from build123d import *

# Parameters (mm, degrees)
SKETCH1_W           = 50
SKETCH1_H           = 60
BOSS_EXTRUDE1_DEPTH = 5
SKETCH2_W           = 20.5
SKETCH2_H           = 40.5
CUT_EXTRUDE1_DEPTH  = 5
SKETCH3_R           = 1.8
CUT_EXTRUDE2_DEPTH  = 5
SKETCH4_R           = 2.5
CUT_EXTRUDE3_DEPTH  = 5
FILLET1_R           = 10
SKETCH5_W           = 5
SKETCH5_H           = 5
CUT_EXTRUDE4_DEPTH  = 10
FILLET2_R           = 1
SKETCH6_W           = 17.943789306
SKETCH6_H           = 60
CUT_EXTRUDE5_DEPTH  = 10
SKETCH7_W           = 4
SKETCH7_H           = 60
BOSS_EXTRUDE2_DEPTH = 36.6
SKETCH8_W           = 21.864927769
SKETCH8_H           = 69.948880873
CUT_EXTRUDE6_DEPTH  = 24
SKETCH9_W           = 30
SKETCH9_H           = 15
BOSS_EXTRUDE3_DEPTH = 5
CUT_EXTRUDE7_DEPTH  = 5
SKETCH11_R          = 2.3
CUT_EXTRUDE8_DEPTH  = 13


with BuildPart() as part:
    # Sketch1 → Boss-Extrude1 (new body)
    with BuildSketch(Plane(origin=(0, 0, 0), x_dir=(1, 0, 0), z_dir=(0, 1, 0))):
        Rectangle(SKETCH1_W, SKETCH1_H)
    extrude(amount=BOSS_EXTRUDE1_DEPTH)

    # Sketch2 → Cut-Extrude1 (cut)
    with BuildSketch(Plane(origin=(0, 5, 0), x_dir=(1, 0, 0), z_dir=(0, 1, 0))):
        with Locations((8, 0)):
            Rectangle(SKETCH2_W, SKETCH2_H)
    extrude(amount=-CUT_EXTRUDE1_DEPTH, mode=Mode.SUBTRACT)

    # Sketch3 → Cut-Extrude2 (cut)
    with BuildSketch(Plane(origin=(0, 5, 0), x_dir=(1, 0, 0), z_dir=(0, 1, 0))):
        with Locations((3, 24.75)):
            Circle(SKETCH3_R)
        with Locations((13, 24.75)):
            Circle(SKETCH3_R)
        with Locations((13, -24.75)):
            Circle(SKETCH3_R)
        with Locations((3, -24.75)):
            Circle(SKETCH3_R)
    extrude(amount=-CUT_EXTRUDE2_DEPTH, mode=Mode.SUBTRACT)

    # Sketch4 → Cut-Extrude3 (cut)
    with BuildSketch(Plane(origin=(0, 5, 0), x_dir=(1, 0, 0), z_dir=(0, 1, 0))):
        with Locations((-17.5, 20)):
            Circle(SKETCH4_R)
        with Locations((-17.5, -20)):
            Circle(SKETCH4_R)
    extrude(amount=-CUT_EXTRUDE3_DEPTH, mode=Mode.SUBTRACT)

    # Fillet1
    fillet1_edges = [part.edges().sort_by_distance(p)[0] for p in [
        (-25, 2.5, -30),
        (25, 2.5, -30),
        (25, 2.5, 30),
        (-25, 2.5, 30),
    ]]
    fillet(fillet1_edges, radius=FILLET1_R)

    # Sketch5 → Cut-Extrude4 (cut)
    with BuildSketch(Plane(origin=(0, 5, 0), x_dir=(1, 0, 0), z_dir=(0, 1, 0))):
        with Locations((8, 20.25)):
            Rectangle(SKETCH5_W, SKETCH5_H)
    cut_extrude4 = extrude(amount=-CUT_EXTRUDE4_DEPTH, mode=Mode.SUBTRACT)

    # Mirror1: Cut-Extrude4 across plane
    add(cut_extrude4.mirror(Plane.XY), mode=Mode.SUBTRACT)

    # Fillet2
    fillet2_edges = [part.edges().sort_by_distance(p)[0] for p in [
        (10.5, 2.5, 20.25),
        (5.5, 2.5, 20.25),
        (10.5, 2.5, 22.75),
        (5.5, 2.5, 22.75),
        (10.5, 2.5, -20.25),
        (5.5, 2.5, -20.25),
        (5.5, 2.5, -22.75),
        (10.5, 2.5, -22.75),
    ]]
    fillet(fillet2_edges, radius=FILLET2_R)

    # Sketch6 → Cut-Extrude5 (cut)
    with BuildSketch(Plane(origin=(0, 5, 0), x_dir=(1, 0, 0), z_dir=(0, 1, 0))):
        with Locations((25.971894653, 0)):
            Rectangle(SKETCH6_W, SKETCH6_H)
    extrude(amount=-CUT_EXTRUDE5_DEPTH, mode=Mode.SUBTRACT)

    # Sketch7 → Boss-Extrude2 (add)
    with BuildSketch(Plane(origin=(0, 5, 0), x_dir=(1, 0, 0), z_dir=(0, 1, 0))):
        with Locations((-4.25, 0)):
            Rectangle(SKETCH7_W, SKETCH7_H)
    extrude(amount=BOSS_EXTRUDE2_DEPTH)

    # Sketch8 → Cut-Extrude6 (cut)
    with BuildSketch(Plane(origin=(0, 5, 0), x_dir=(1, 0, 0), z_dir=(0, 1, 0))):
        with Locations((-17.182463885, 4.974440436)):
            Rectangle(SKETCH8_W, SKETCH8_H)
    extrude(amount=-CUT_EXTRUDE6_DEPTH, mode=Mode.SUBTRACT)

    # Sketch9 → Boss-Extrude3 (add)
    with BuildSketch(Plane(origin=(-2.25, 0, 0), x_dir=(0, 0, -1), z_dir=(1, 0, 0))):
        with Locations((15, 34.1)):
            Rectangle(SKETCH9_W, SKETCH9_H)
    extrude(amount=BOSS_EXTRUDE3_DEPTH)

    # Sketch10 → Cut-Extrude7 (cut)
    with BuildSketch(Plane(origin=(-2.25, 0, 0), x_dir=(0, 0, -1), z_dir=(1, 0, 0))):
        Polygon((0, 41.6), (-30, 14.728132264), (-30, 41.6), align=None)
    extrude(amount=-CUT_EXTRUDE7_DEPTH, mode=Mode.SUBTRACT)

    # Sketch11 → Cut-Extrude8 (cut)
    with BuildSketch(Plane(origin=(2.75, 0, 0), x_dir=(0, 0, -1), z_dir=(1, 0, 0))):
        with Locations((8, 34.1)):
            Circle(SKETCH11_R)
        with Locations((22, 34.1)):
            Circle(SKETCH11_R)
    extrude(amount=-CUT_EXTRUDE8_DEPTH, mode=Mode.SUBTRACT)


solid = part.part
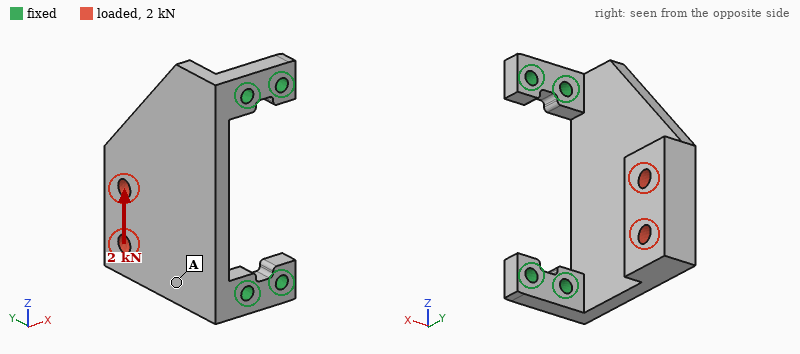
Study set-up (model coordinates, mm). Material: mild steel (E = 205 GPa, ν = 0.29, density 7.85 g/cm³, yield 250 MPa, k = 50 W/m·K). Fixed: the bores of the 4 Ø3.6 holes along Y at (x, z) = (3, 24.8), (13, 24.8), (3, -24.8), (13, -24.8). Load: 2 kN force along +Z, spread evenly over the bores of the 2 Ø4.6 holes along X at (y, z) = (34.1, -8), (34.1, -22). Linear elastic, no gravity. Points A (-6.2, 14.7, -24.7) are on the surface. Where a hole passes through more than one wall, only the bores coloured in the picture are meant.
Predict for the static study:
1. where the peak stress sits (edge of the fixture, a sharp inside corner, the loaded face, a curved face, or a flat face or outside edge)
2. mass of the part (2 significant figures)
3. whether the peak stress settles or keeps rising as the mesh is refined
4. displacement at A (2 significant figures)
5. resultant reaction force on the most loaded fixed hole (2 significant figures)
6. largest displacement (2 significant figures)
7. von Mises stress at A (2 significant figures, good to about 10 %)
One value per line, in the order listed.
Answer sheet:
edge of the fixture
93 g
keeps rising
19 µm
1.8 kN
50 µm
35 MPa
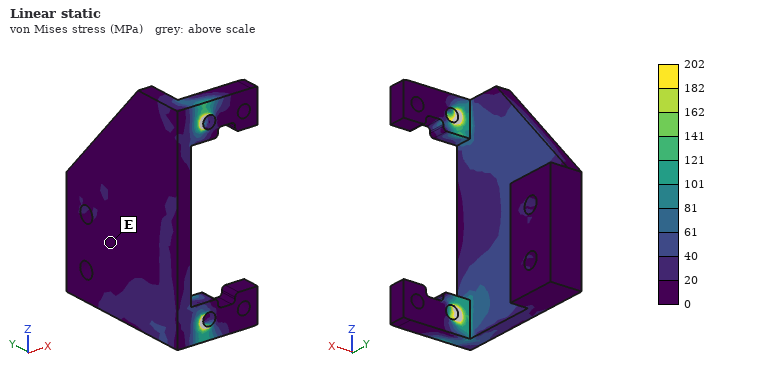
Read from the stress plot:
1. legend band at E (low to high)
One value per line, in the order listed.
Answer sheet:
0 to 20 MPa
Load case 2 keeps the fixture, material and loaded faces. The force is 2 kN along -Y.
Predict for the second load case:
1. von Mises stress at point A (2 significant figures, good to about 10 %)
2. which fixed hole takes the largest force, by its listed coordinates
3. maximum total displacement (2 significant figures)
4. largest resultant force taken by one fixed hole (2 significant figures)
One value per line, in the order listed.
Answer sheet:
26 MPa
(3, -24.8)
64 µm
1.7 kN
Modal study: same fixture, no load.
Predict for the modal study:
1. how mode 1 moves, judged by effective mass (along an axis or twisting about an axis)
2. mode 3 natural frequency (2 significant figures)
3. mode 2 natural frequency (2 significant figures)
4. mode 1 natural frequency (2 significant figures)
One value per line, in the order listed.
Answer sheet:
along X
7000 Hz
4400 Hz
1200 Hz
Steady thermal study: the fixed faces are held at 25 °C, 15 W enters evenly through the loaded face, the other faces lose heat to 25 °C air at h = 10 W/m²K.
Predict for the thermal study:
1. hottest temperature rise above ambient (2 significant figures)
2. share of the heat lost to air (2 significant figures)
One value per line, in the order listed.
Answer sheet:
75 K
16 %
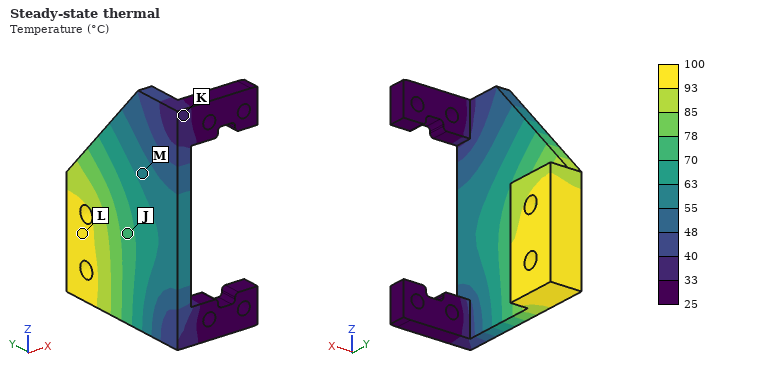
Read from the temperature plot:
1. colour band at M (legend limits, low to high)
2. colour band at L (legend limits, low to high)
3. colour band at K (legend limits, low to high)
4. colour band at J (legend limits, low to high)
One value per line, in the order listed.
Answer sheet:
55 to 63 °C
93 to 100 °C
33 to 40 °C
70 to 78 °C
